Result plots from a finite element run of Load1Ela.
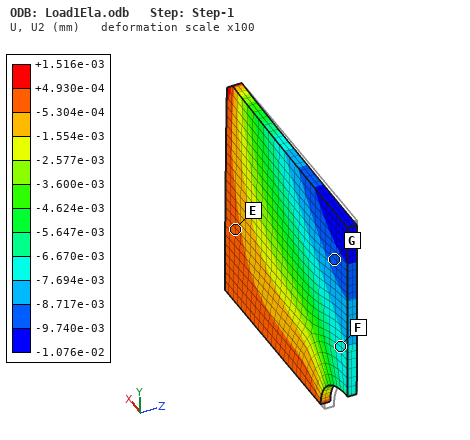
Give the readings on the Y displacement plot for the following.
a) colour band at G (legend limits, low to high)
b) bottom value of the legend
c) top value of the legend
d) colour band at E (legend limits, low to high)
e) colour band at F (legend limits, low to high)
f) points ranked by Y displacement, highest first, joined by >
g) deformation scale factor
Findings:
-9.740e-03 to -8.717e-03 mm
-1.076e-02 mm
+1.516e-03 mm
-5.304e-04 to +4.930e-04 mm
-7.694e-03 to -6.670e-03 mm
E > F > G
100
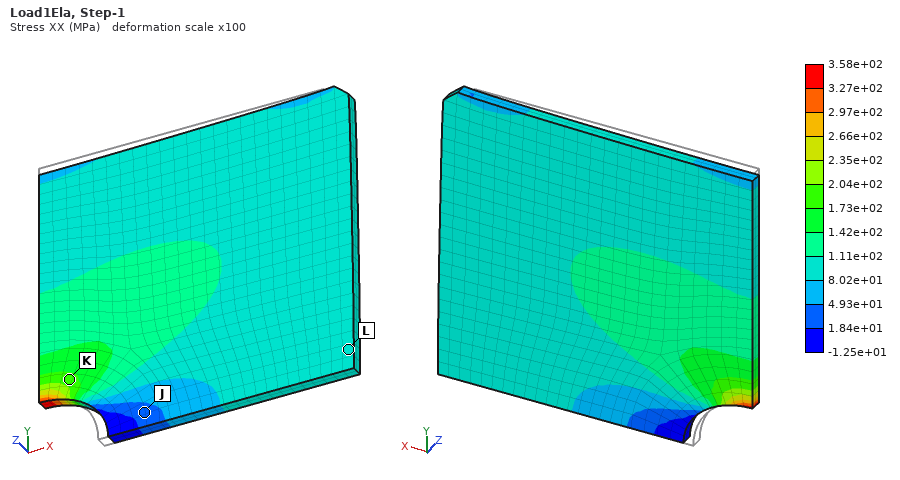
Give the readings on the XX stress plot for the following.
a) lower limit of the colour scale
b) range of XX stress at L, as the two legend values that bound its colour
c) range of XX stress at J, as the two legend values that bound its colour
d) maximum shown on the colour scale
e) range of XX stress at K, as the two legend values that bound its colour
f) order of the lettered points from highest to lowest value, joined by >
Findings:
-1.25e+01 MPa
8.02e+01 to 1.11e+02 MPa
1.84e+01 to 4.93e+01 MPa
3.58e+02 MPa
1.73e+02 to 2.04e+02 MPa
K > L > J
